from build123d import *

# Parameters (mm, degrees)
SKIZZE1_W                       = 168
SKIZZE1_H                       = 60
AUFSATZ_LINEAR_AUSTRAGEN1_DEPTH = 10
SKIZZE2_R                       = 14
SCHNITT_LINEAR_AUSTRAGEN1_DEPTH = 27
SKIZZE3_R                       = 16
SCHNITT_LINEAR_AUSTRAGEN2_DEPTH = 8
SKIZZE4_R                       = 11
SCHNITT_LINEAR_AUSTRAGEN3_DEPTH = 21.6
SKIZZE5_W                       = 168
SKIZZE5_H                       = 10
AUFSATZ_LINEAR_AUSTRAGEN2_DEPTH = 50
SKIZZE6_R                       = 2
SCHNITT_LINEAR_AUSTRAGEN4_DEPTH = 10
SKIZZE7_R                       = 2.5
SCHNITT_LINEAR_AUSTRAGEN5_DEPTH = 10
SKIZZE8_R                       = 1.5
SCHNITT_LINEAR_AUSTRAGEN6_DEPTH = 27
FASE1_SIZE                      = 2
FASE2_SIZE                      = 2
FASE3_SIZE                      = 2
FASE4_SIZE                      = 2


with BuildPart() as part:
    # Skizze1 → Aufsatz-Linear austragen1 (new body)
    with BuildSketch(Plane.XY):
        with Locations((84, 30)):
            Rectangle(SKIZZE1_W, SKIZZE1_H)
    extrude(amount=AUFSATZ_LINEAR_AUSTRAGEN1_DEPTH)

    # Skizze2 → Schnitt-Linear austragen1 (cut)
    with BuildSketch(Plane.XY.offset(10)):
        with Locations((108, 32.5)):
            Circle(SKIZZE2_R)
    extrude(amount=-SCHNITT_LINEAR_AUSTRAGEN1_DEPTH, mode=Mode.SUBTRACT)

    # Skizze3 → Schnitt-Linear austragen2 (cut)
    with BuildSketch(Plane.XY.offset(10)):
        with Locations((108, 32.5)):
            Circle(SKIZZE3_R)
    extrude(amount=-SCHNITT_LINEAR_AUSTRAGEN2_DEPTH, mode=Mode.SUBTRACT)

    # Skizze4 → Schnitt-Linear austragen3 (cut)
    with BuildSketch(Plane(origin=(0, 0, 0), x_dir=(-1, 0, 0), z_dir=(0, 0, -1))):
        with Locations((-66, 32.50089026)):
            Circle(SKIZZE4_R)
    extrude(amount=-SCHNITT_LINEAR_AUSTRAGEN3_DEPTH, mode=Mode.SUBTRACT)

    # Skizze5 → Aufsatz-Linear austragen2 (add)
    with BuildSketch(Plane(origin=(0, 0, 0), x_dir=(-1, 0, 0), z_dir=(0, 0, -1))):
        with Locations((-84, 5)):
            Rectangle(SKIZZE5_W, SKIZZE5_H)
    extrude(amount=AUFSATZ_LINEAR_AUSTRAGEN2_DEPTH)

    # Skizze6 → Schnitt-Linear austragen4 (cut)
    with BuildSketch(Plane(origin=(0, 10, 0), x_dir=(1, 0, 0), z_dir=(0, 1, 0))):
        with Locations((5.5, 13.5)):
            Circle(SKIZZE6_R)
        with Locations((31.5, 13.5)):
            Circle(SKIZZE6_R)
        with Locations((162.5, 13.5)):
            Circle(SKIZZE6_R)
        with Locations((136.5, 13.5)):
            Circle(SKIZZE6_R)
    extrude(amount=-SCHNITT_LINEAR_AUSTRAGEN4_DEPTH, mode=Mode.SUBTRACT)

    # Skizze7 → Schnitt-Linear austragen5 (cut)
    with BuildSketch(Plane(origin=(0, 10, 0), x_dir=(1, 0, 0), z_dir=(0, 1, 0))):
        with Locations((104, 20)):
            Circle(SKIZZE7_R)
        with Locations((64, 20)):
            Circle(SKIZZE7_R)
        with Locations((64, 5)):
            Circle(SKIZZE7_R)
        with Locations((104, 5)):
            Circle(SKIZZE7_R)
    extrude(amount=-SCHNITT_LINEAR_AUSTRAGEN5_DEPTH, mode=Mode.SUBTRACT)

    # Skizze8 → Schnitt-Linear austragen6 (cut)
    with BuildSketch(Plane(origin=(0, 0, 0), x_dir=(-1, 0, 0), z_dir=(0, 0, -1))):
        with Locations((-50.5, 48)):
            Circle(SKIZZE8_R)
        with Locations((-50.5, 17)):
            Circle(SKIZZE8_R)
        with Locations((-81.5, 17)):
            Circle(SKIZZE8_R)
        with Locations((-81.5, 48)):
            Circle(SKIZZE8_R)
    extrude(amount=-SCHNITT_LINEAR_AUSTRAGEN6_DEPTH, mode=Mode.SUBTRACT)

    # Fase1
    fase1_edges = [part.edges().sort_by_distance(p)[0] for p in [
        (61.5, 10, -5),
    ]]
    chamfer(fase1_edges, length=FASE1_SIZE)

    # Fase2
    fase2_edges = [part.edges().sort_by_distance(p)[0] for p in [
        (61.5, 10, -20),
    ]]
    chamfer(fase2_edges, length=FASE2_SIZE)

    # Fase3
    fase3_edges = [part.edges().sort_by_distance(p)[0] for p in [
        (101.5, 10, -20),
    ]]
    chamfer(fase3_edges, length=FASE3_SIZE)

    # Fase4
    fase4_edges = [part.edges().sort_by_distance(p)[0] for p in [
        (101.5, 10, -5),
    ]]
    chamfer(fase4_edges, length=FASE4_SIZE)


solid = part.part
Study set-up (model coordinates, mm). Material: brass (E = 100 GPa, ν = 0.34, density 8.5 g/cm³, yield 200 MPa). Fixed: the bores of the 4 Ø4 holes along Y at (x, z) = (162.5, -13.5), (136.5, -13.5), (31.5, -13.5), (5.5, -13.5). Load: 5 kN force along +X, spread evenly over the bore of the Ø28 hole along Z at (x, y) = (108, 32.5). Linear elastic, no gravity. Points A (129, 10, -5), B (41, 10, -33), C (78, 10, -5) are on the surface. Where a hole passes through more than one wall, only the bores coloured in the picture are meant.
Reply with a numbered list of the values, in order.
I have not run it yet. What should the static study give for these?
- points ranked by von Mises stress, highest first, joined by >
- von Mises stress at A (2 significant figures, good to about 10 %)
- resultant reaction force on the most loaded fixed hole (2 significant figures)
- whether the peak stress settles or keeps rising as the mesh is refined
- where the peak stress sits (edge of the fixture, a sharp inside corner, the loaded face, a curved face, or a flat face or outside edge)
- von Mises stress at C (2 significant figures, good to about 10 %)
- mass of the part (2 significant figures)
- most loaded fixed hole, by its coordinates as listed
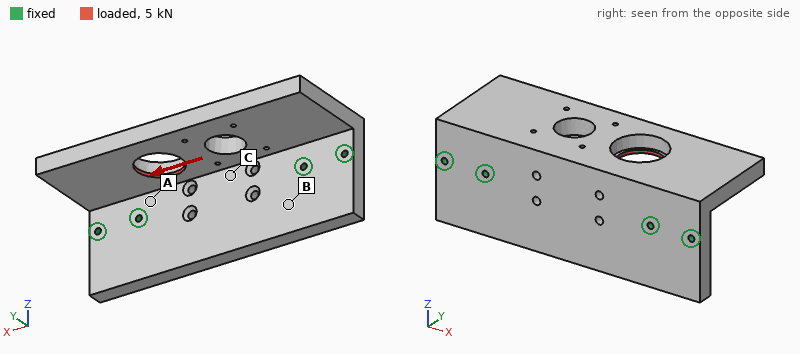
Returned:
1. A > C > B
2. 15 MPa
3. 1.9 kN
4. keeps rising
5. edge of the fixture
6. 8.8 MPa
7. 1.5 kg
8. (136.5, -13.5)
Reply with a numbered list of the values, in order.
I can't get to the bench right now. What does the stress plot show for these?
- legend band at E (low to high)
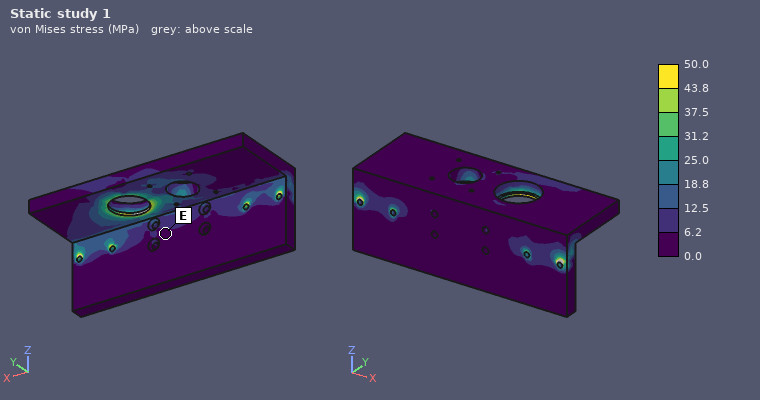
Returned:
1. 0.0 to 6.2 MPa
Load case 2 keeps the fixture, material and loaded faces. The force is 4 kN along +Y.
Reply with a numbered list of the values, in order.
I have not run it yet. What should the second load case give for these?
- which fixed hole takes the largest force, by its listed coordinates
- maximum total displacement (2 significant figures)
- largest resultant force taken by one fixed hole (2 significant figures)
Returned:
1. (136.5, -13.5)
2. 42 µm
3. 2.1 kN
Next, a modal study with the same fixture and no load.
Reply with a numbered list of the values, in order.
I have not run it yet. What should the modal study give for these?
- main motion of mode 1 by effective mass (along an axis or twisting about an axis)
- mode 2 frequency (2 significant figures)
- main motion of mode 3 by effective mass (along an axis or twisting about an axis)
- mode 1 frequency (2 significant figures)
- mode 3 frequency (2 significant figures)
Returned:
1. along Z
2. 1600 Hz
3. along Y
4. 1000 Hz
5. 2400 Hz
